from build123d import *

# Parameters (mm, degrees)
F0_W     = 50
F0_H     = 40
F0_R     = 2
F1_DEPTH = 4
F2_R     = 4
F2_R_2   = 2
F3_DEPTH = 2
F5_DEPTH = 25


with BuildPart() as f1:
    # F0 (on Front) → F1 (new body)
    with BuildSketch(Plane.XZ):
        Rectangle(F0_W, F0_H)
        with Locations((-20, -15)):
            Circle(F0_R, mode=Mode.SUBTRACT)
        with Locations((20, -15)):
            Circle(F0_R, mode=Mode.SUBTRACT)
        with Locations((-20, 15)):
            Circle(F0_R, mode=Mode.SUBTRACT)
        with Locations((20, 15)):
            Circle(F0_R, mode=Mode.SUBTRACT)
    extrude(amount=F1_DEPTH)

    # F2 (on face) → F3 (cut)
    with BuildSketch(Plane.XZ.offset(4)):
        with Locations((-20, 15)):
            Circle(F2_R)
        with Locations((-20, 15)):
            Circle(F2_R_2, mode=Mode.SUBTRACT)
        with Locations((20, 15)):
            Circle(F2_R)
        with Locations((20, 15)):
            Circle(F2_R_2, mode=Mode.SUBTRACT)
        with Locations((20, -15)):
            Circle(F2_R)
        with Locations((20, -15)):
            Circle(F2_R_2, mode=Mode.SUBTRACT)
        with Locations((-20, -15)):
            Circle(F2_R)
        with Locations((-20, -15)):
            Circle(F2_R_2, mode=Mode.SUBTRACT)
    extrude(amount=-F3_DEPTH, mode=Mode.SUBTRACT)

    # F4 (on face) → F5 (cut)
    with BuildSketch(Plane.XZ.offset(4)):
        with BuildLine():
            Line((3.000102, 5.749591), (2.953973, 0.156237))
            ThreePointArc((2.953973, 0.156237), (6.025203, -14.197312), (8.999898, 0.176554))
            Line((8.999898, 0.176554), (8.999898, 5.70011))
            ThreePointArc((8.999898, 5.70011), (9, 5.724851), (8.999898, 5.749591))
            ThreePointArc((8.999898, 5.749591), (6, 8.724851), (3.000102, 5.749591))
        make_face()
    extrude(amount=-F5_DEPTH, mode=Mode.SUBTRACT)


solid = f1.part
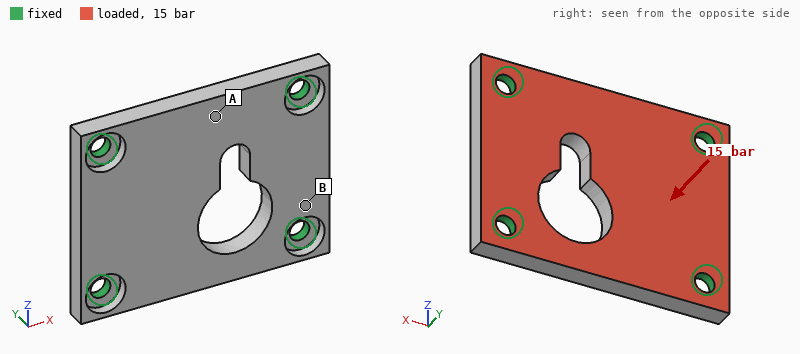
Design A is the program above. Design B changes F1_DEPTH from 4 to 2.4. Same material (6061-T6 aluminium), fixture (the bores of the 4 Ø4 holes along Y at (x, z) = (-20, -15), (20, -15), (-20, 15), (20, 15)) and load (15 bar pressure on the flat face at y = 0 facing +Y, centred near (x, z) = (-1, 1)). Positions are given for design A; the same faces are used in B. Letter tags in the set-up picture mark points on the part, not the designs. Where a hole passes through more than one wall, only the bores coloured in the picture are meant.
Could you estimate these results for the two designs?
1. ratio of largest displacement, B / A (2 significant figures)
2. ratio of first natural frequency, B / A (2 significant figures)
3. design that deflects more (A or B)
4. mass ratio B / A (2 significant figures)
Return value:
3.0
0.77
B
0.62
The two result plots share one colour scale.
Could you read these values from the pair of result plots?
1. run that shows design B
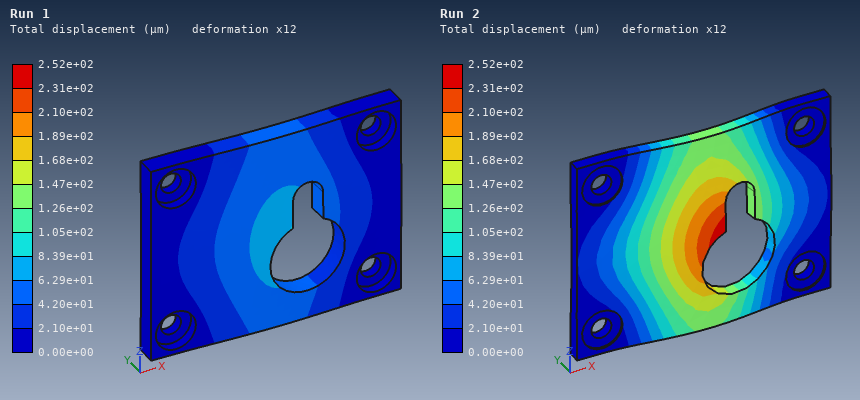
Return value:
Run 2
